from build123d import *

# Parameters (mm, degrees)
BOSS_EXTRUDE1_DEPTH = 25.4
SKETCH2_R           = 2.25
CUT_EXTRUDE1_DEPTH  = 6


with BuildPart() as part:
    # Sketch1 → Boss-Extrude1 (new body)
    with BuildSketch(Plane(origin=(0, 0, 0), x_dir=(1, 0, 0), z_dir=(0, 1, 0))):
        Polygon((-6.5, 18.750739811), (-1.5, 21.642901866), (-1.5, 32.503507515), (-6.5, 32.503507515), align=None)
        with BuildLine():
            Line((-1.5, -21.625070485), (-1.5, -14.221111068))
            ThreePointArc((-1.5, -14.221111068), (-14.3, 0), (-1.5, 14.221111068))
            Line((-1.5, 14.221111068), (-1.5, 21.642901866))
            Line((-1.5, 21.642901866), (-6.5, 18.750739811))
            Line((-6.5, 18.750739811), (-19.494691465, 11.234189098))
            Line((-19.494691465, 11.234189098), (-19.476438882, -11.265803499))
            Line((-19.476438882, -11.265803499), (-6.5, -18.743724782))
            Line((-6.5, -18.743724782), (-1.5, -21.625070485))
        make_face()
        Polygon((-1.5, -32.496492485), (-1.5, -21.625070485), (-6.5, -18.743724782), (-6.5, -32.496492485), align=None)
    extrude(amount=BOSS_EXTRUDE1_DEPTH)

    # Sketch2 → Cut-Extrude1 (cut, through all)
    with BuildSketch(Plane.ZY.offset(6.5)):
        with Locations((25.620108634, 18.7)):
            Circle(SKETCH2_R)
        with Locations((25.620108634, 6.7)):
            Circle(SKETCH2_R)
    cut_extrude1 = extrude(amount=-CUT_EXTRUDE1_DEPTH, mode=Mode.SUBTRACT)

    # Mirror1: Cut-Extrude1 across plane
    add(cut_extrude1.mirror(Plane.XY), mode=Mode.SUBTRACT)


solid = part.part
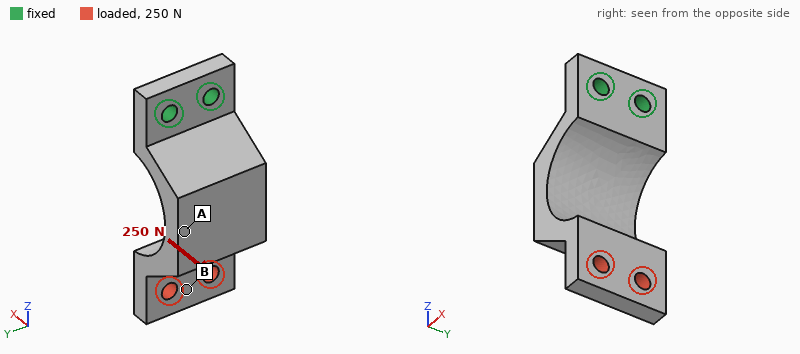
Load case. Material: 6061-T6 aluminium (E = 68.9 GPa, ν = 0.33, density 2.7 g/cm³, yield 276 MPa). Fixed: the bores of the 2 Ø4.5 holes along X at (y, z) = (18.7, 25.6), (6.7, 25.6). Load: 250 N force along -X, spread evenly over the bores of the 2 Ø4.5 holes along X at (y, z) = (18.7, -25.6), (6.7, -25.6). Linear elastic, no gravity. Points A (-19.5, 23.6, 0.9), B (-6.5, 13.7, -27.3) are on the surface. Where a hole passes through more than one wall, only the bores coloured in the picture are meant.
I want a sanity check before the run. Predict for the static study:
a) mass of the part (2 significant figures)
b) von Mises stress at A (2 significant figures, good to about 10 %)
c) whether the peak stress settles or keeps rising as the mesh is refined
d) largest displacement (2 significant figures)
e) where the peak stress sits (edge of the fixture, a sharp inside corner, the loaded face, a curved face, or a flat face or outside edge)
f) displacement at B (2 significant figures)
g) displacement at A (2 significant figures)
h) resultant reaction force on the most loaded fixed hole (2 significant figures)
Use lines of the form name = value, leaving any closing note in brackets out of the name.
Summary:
mass of the part = 29 g
von Mises stress at A = 56 MPa
whether the peak stress settles or keeps rising as the mesh is refined = keeps rising
largest displacement = 0.65 mm
where the peak stress sits = edge of the fixture
displacement at B = 0.56 mm
displacement at A = 0.20 mm
resultant reaction force on the most loaded fixed hole = 140 N
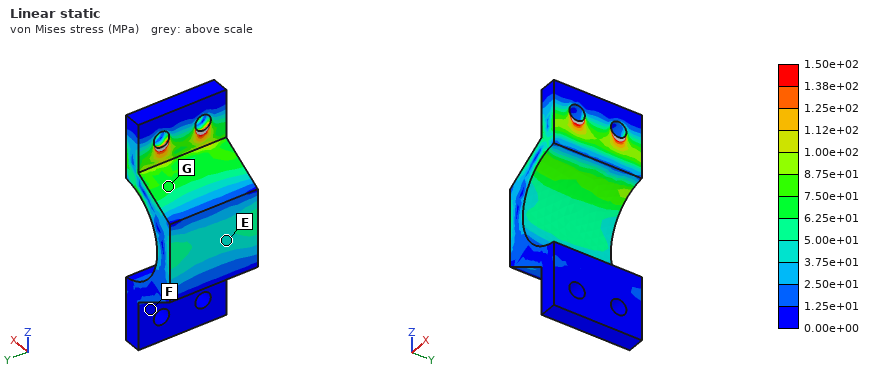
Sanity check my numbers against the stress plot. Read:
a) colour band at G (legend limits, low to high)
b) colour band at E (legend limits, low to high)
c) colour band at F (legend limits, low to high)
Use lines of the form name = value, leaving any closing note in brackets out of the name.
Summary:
colour band at G = 6.25e+01 to 7.50e+01 MPa
colour band at E = 3.75e+01 to 5.00e+01 MPa
colour band at F = 0.00e+00 to 1.25e+01 MPa
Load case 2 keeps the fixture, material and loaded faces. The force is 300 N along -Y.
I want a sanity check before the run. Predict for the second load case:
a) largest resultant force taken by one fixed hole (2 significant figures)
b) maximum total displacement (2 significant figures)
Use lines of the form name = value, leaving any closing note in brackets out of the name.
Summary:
largest resultant force taken by one fixed hole = 1.0 kN
maximum total displacement = 0.20 mm
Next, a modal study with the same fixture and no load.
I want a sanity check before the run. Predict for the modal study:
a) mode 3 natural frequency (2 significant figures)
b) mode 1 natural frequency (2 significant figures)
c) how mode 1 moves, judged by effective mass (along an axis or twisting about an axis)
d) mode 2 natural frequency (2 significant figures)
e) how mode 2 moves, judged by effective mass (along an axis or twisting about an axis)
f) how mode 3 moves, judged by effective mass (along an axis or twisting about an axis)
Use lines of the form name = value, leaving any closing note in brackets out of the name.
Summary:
mode 3 natural frequency = 4400 Hz
mode 1 natural frequency = 1200 Hz
how mode 1 moves, judged by effective mass = along X
mode 2 natural frequency = 2400 Hz
how mode 2 moves, judged by effective mass = along Y
how mode 3 moves, judged by effective mass = along Z
